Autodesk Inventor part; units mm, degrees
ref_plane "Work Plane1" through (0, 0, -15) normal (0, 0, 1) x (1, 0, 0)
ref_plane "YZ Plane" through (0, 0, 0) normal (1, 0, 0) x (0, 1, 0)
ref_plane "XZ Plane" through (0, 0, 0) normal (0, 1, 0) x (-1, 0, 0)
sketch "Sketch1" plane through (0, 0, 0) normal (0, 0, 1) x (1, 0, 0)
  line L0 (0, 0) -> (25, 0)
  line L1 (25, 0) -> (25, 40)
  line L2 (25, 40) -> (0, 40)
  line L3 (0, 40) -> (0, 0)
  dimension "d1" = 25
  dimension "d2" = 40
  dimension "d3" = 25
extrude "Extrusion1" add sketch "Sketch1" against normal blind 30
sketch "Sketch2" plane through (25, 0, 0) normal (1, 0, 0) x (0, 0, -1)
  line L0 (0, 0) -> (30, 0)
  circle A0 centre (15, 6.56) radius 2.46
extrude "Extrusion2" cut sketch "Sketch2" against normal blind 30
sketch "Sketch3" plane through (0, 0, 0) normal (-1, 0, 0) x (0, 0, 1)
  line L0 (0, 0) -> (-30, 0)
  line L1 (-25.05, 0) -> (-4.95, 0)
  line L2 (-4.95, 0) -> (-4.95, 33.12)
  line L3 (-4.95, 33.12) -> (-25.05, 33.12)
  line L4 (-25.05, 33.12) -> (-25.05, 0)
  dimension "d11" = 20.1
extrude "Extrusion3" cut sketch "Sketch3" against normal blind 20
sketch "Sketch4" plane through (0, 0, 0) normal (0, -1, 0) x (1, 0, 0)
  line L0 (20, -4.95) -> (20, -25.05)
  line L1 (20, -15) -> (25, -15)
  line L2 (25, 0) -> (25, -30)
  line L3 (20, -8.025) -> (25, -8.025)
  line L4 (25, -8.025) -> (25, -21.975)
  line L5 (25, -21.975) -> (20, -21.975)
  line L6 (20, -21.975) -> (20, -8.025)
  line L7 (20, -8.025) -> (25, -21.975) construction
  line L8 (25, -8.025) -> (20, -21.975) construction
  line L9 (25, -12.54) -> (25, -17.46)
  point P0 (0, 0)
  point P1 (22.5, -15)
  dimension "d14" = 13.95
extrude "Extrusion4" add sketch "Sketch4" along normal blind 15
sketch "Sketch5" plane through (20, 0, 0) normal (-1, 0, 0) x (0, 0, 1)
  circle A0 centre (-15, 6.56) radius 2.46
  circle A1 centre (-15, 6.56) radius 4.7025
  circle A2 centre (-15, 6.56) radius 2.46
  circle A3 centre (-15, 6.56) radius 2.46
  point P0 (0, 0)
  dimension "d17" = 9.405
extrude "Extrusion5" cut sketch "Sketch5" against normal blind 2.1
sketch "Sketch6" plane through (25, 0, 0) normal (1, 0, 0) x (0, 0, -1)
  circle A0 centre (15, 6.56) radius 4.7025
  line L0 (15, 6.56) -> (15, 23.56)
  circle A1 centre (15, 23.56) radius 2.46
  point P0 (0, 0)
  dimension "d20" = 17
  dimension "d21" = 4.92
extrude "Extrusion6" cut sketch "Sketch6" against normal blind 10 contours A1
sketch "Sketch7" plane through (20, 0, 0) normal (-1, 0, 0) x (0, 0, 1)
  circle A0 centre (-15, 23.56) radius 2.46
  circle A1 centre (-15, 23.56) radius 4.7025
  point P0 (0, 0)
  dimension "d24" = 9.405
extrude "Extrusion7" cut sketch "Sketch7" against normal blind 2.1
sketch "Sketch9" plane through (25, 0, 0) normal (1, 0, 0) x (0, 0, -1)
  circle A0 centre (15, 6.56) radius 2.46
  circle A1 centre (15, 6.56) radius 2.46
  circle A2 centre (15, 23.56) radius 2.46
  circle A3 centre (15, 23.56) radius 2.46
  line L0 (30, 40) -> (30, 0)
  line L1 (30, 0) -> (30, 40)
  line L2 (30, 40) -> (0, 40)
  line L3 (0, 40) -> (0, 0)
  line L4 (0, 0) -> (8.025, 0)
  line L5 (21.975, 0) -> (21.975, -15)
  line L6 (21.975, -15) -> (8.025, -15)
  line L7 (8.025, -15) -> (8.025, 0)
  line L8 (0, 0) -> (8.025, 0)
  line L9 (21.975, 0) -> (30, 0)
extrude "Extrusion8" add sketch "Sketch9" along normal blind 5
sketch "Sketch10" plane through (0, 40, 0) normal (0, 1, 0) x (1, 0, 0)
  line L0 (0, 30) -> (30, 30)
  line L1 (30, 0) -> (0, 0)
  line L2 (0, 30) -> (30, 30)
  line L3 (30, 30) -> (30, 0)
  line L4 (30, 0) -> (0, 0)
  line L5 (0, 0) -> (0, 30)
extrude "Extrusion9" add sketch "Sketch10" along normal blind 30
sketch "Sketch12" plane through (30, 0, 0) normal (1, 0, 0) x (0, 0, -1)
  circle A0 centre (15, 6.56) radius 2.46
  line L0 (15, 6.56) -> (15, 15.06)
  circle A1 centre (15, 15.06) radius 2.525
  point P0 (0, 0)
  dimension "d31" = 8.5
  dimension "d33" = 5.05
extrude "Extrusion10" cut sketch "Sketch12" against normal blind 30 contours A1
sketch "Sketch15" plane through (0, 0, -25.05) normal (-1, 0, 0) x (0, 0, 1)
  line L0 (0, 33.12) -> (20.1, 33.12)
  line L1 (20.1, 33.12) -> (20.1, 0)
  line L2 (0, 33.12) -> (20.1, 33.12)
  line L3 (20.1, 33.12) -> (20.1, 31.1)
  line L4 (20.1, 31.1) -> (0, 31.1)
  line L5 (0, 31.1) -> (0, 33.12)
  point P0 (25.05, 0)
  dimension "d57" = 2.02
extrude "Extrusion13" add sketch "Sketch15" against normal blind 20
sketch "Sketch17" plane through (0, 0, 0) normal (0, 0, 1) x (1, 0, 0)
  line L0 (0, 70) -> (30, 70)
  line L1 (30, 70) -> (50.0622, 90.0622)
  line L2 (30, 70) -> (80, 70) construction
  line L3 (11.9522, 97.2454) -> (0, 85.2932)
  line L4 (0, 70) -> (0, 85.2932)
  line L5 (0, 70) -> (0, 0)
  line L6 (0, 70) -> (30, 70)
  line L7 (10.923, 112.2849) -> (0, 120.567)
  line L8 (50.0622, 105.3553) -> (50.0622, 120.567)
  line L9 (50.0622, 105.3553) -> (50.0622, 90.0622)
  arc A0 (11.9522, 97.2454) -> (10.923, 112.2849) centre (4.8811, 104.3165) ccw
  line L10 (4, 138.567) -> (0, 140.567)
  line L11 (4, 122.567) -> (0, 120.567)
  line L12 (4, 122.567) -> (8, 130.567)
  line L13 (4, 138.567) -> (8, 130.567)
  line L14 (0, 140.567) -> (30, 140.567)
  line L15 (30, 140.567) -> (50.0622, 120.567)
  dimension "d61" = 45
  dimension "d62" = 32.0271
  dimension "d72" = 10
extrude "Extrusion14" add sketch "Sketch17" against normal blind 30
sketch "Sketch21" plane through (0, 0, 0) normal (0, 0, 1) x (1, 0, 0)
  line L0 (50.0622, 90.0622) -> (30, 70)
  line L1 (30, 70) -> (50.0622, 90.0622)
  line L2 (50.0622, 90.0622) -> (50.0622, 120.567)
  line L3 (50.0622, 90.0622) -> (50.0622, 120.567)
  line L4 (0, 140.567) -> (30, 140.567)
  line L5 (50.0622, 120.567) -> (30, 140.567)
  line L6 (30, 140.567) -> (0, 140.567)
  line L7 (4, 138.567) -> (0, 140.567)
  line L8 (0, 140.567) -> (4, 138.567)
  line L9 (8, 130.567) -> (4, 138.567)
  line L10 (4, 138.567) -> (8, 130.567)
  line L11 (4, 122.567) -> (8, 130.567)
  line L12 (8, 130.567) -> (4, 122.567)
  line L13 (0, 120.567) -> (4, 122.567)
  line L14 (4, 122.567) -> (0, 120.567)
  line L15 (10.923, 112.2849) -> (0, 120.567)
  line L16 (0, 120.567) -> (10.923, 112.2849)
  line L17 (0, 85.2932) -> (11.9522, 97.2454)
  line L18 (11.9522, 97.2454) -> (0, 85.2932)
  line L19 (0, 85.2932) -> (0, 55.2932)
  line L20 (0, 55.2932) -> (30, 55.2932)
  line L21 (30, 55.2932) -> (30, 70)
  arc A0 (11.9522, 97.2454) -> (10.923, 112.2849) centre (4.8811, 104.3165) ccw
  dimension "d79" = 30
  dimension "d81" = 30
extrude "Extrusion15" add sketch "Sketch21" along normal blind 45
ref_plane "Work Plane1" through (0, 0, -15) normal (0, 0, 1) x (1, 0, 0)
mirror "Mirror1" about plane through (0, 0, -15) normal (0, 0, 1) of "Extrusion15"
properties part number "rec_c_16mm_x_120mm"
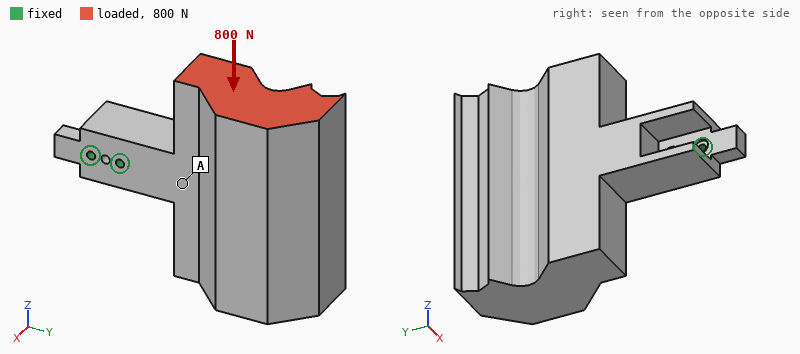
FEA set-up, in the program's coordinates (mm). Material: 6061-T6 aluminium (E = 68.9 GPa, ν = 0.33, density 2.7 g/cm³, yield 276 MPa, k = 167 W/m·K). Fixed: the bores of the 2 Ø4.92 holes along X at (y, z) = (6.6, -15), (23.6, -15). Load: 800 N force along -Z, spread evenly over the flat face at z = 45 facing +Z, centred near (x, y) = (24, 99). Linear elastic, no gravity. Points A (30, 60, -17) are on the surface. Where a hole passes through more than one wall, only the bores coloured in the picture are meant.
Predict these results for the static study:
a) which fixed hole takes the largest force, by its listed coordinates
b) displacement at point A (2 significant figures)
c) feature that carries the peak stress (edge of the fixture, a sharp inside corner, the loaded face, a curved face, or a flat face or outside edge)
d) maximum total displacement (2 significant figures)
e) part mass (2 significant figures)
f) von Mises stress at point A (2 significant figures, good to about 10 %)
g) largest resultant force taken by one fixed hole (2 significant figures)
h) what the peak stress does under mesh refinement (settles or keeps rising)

(23.6, -15)
0.042 mm
edge of the fixture
0.16 mm
1.1 kg
5.5 MPa
3.4 kN
keeps rising
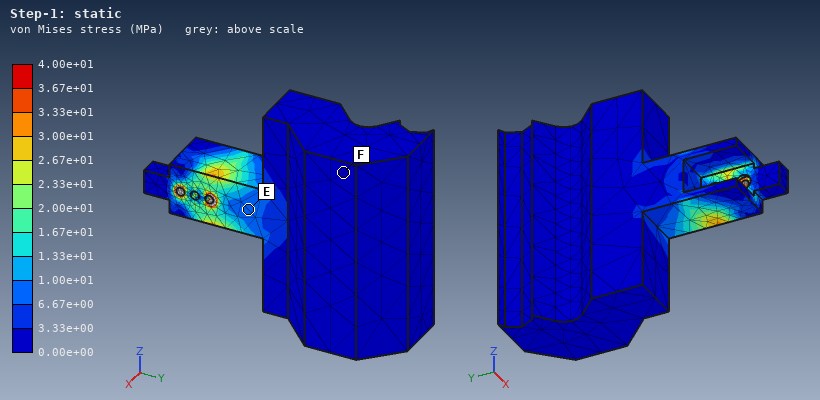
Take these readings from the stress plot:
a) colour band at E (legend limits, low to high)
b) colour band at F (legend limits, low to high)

6.67e+00 to 1.00e+01 MPa
0.00e+00 to 3.33e+00 MPa
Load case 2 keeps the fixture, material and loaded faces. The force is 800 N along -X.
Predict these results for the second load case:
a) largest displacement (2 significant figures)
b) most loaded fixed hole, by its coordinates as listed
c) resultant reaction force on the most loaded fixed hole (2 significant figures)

0.36 mm
(23.6, -15)
3.2 kN
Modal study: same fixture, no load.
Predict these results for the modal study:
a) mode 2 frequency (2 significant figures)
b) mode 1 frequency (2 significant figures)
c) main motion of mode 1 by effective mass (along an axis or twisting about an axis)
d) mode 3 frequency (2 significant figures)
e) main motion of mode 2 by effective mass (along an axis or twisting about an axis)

400 Hz
380 Hz
along X
580 Hz
along Z
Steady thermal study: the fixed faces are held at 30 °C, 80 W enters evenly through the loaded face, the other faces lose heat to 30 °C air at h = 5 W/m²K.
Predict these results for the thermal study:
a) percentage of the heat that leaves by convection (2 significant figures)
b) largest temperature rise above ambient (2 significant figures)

8.8 %
45 K
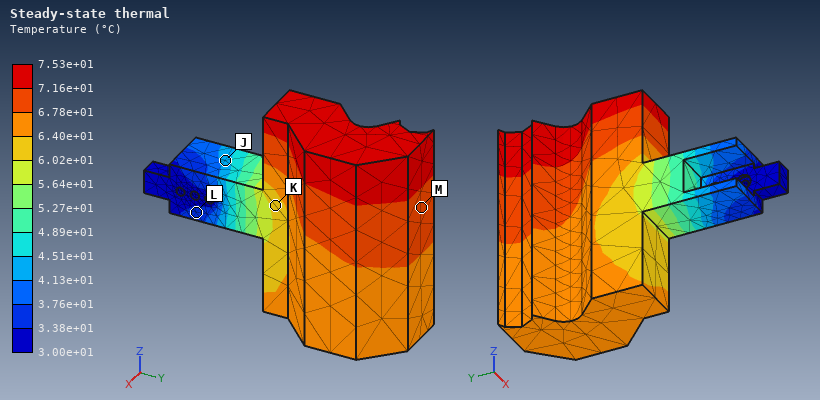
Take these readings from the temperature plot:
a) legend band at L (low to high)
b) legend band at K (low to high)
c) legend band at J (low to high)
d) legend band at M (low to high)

3.38e+01 to 3.76e+01 °C
6.02e+01 to 6.40e+01 °C
4.13e+01 to 4.51e+01 °C
6.78e+01 to 7.16e+01 °C
